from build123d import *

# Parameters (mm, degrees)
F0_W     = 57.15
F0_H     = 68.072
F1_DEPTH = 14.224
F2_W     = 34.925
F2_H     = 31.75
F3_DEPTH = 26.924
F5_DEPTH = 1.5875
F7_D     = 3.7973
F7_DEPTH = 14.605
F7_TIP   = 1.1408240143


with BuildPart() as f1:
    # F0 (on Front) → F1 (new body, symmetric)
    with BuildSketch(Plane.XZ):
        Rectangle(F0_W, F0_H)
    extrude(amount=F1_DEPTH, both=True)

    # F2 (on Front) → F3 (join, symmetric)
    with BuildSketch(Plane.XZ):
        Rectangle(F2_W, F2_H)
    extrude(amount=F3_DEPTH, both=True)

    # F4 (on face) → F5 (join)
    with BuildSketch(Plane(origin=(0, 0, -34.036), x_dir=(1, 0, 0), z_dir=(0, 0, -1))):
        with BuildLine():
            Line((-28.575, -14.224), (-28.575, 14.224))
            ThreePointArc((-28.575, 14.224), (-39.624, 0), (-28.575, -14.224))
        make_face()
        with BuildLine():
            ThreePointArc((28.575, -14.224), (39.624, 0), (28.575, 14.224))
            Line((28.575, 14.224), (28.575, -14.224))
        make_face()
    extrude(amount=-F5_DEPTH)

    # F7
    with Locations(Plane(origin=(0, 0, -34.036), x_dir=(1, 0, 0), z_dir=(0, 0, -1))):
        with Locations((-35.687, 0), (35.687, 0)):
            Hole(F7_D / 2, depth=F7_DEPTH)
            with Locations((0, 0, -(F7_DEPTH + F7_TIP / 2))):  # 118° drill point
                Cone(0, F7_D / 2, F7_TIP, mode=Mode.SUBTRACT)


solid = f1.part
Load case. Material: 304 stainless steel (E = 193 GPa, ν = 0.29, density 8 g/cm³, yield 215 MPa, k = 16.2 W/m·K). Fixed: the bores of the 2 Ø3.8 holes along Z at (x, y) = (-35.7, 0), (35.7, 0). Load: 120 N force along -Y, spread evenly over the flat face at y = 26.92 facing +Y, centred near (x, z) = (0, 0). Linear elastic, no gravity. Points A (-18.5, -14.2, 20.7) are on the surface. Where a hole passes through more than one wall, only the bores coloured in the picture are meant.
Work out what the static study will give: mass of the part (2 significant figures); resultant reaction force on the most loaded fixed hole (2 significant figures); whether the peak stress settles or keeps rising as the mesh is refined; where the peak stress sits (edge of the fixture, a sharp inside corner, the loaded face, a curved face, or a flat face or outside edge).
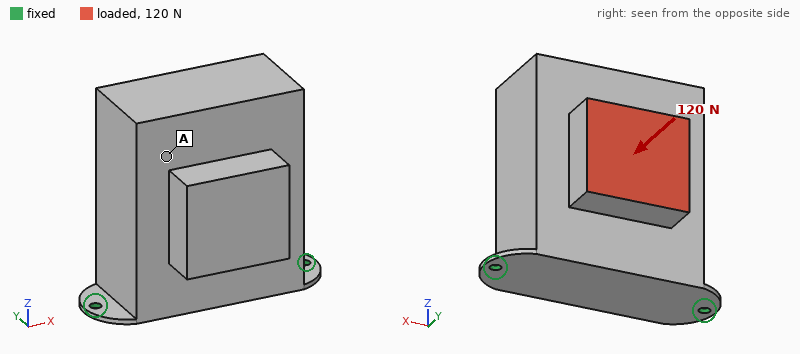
1.1 kg
60 N
keeps rising
edge of the fixture
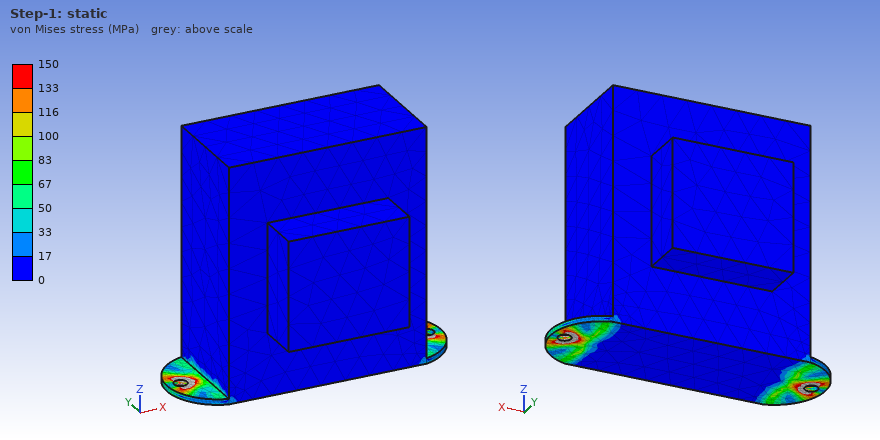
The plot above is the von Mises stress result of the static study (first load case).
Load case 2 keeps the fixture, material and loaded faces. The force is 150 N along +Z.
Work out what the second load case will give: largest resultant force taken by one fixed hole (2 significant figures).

84 N
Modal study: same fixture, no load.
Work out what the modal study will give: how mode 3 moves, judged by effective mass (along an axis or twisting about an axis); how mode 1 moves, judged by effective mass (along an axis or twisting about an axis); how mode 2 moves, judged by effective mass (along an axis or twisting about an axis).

along Z
along Y
along X
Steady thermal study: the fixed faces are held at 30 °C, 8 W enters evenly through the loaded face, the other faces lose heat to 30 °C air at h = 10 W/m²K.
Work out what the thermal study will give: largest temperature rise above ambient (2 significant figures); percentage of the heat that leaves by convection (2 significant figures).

40 K
67 %
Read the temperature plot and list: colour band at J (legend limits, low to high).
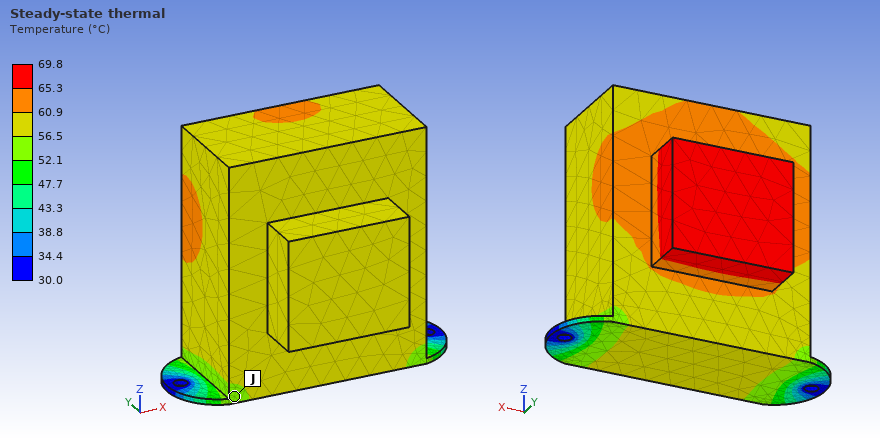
52.1 to 56.5 °C
